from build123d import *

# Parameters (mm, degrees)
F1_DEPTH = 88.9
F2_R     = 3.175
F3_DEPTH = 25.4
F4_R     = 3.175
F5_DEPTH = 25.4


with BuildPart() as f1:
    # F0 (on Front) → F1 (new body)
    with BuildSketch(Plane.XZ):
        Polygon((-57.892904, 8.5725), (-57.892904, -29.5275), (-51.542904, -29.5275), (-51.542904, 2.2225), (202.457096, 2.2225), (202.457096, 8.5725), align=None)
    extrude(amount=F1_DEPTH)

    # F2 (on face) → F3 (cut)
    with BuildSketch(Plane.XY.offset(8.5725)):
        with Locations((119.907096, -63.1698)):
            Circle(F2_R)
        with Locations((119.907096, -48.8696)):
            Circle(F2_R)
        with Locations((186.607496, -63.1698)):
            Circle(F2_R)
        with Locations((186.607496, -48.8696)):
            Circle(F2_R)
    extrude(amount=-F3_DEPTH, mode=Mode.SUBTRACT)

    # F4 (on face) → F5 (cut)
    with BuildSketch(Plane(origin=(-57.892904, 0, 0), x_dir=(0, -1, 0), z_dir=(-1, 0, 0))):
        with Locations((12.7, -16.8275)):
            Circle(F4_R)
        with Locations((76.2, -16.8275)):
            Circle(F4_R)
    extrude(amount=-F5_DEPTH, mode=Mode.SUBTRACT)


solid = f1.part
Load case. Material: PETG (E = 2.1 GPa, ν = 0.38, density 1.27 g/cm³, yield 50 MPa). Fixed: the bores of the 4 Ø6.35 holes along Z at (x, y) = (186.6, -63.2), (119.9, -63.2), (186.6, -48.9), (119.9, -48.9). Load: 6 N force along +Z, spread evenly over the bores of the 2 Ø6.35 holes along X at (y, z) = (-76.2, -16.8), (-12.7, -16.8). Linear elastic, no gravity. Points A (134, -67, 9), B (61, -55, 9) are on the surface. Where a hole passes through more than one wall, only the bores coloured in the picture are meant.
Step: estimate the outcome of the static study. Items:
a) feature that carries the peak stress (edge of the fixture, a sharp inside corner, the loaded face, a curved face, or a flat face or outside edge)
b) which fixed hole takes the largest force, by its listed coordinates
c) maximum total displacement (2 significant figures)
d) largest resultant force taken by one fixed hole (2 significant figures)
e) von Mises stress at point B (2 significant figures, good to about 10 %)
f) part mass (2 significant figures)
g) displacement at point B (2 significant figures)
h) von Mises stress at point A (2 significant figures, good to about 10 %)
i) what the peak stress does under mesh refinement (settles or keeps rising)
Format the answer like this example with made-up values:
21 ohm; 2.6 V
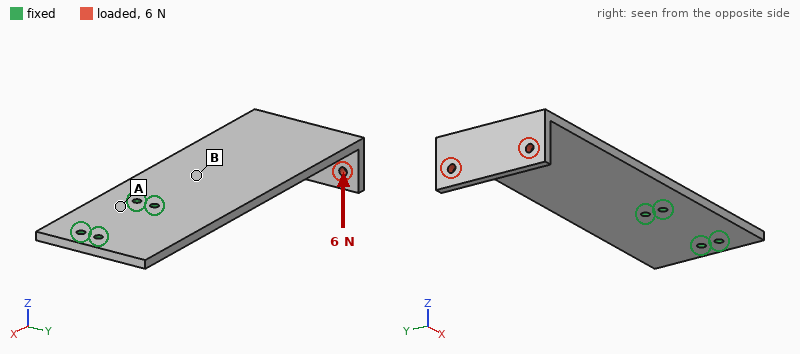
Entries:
edge of the fixture; (119.9, -48.9); 2.9 mm; 11 N; 1.1 MPa; 210 g; 0.44 mm; 0.31 MPa; keeps rising
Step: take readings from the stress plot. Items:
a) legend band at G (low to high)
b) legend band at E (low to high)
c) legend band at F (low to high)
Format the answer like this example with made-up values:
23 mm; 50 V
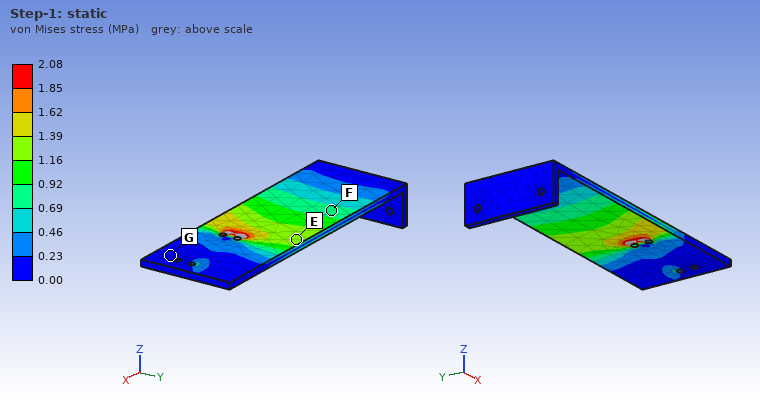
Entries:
0.00 to 0.23 MPa; 1.16 to 1.39 MPa; 0.69 to 0.92 MPa
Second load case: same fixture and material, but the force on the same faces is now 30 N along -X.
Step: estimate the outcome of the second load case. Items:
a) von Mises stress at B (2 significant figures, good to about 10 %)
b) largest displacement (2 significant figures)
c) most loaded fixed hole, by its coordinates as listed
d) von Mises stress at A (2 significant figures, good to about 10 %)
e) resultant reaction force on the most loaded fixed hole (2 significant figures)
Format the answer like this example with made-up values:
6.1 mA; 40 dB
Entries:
1.0 MPa; 2.8 mm; (119.9, -48.9); 0.23 MPa; 16 N
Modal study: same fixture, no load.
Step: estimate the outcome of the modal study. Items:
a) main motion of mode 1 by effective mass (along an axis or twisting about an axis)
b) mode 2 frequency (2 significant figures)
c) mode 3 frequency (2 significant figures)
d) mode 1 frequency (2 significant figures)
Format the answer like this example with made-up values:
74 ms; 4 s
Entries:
along Z; 120 Hz; 200 Hz; 32 Hz
